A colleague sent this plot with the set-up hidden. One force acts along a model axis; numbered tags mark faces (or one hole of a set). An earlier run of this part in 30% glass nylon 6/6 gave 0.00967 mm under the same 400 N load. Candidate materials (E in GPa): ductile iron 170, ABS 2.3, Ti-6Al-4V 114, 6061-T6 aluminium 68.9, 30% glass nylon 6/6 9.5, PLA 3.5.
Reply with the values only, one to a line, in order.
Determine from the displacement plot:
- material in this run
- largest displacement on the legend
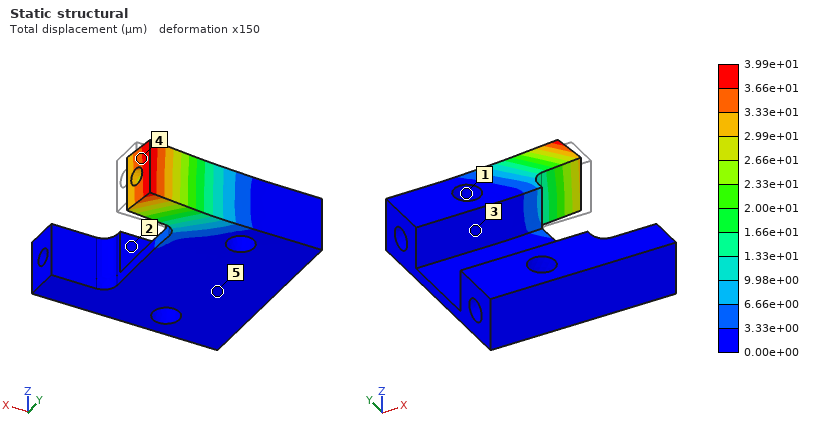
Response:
ABS
3.99e+01 µm
